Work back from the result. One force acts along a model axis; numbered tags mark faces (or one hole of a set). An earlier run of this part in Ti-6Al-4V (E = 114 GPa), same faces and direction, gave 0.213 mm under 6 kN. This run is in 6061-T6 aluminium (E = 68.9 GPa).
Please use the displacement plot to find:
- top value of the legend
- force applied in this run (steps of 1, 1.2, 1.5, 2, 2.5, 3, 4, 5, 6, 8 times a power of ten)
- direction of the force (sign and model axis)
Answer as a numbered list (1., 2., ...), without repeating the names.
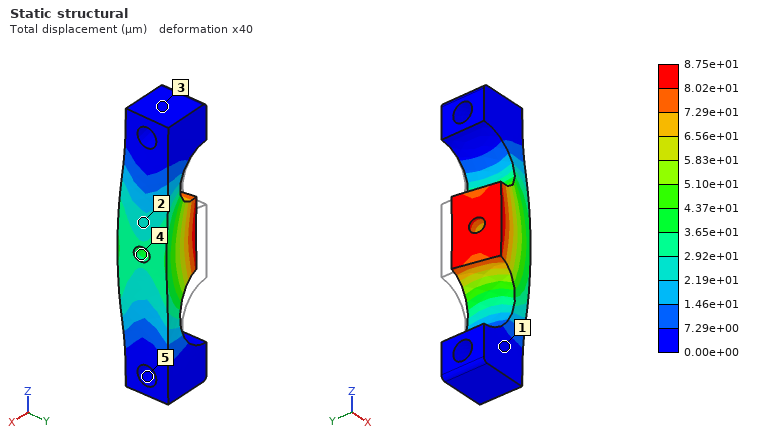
1. 8.75e+01 µm
2. 1.5 kN
3. -Y
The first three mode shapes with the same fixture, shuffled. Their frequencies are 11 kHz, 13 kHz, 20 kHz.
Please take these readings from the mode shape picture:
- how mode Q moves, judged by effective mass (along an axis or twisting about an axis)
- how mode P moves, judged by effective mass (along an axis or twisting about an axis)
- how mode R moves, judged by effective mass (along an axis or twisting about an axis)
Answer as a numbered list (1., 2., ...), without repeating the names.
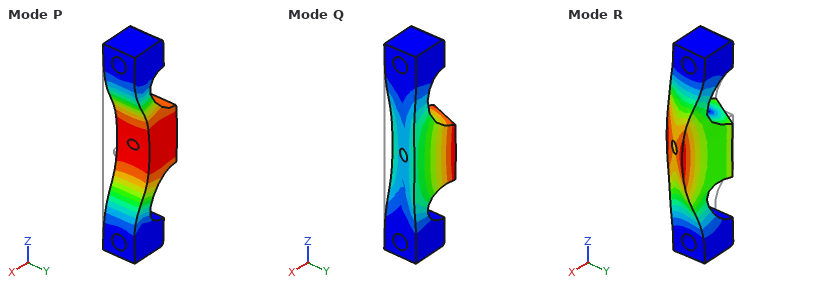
1. along Y
2. along X
3. along Y
